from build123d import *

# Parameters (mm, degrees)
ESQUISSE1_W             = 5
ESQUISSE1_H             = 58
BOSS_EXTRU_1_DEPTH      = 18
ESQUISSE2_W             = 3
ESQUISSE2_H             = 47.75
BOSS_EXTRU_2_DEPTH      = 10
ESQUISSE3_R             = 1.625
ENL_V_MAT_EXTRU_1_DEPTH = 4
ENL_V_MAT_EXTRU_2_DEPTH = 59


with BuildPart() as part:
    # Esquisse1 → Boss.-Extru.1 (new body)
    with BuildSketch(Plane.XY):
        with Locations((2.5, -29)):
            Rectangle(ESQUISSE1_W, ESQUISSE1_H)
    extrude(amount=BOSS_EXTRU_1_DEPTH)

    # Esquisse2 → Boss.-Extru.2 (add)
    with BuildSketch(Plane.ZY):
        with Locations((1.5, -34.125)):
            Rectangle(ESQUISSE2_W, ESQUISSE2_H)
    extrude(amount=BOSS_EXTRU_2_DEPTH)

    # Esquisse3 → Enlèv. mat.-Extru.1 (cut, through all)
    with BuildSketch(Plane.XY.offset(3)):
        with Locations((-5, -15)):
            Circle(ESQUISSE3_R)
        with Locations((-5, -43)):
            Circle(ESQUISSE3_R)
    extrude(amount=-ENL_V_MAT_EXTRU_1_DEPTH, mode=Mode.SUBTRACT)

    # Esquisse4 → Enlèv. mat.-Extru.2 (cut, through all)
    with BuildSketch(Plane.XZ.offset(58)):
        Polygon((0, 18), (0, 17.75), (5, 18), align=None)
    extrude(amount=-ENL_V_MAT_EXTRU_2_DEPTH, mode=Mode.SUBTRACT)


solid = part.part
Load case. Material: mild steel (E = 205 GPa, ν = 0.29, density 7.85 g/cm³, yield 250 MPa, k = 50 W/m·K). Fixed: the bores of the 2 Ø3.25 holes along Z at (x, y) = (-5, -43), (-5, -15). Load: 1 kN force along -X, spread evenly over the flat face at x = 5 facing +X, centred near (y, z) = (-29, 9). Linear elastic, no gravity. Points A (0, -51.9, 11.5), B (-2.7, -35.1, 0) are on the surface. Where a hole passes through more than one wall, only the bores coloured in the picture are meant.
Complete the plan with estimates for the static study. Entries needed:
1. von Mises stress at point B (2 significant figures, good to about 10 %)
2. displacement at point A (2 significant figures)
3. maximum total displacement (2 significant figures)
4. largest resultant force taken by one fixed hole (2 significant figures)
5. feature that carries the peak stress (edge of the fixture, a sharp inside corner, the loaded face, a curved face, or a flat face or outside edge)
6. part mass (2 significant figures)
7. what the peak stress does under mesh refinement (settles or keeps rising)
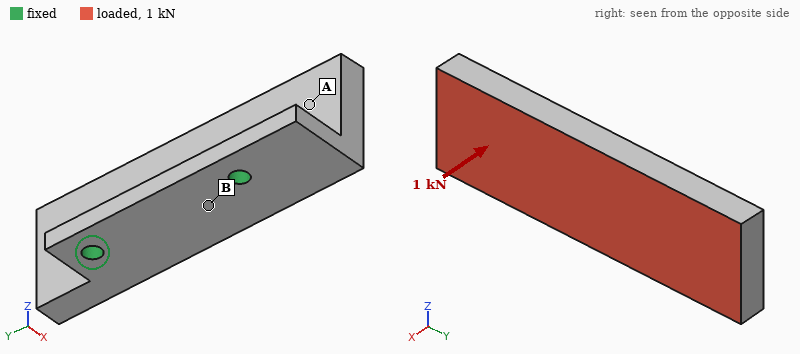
62 MPa
29 µm
60 µm
510 N
edge of the fixture
52 g
keeps rising
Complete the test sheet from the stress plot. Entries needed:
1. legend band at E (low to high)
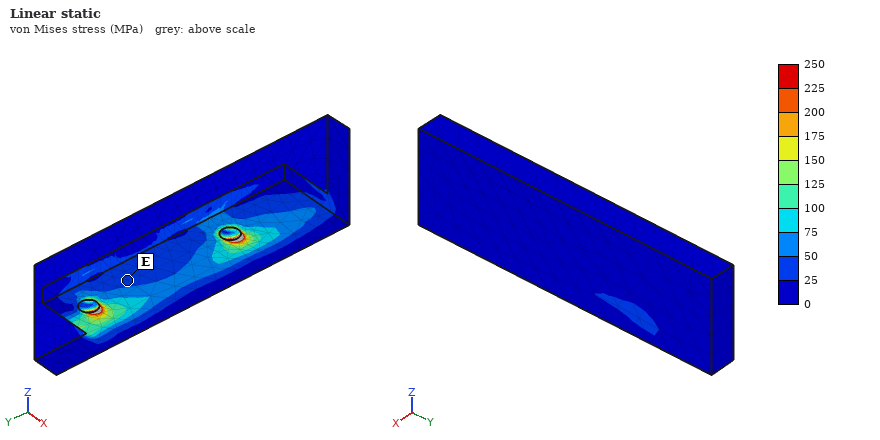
25 to 50 MPa
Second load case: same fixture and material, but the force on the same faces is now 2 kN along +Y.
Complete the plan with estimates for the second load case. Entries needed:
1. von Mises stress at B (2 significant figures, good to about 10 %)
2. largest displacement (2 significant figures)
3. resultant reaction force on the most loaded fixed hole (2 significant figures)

19 MPa
12 µm
1.3 kN
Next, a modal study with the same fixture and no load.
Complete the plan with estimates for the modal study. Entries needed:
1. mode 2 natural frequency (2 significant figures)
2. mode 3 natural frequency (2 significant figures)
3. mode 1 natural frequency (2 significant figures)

6800 Hz
11 kHz
3900 Hz
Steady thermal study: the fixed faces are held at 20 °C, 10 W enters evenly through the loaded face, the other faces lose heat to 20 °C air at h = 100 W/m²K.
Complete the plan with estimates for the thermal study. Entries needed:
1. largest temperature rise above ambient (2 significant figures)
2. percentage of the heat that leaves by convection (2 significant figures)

16 K
28 %
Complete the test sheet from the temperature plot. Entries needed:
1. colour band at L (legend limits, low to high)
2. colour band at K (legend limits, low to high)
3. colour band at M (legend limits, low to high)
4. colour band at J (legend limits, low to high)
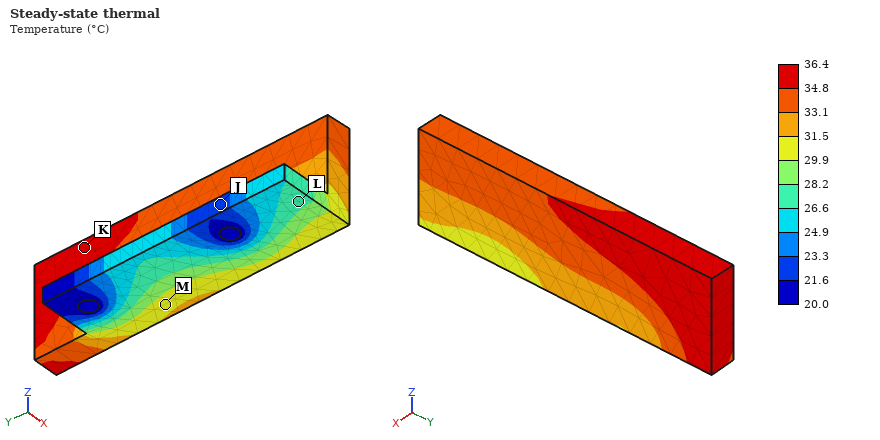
26.6 to 28.2 °C
34.8 to 36.4 °C
29.9 to 31.5 °C
21.6 to 23.3 °C
